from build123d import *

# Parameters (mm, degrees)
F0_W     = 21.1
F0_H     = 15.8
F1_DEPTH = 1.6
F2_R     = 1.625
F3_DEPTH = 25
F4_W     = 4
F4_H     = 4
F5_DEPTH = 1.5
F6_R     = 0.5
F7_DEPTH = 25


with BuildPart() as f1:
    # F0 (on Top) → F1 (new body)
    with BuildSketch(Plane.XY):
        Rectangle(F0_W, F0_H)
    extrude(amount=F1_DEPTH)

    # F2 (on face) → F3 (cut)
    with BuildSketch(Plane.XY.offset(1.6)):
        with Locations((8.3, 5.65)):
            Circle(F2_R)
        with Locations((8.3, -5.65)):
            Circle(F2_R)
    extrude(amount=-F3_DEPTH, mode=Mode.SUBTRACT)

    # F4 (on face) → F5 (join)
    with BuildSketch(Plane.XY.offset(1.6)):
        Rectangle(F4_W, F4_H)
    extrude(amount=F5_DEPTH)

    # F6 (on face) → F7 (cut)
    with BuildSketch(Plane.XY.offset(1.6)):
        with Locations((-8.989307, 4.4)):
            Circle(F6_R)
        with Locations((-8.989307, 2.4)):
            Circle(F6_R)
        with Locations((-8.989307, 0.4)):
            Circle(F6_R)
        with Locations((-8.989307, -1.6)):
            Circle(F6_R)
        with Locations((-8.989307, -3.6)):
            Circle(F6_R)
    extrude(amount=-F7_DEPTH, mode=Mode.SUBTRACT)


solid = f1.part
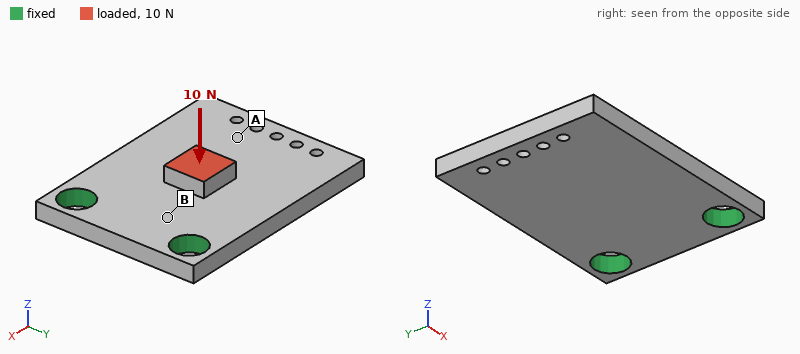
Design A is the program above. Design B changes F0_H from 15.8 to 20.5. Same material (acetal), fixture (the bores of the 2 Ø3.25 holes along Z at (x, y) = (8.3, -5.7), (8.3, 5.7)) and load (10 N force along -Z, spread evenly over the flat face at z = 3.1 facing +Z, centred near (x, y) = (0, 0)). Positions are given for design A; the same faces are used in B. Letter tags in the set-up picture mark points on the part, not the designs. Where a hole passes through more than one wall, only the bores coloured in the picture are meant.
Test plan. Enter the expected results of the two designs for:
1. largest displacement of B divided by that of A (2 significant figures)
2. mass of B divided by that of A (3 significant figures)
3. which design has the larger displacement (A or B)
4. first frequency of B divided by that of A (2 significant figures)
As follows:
0.79
1.30
A
1.00
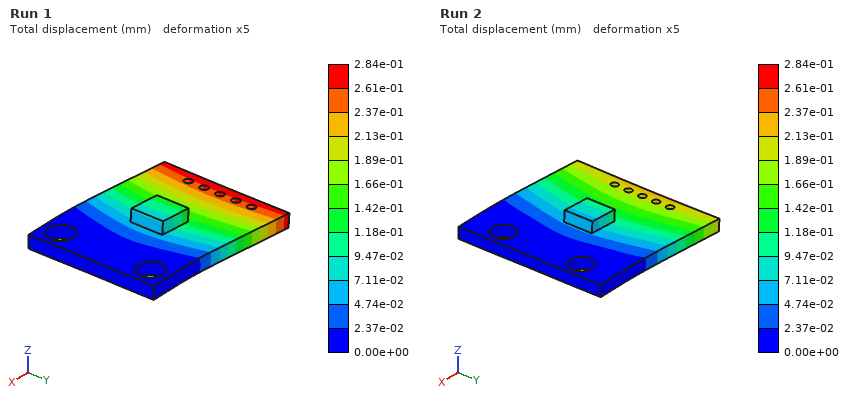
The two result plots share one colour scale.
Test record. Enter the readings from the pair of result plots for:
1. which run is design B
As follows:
Run 2
